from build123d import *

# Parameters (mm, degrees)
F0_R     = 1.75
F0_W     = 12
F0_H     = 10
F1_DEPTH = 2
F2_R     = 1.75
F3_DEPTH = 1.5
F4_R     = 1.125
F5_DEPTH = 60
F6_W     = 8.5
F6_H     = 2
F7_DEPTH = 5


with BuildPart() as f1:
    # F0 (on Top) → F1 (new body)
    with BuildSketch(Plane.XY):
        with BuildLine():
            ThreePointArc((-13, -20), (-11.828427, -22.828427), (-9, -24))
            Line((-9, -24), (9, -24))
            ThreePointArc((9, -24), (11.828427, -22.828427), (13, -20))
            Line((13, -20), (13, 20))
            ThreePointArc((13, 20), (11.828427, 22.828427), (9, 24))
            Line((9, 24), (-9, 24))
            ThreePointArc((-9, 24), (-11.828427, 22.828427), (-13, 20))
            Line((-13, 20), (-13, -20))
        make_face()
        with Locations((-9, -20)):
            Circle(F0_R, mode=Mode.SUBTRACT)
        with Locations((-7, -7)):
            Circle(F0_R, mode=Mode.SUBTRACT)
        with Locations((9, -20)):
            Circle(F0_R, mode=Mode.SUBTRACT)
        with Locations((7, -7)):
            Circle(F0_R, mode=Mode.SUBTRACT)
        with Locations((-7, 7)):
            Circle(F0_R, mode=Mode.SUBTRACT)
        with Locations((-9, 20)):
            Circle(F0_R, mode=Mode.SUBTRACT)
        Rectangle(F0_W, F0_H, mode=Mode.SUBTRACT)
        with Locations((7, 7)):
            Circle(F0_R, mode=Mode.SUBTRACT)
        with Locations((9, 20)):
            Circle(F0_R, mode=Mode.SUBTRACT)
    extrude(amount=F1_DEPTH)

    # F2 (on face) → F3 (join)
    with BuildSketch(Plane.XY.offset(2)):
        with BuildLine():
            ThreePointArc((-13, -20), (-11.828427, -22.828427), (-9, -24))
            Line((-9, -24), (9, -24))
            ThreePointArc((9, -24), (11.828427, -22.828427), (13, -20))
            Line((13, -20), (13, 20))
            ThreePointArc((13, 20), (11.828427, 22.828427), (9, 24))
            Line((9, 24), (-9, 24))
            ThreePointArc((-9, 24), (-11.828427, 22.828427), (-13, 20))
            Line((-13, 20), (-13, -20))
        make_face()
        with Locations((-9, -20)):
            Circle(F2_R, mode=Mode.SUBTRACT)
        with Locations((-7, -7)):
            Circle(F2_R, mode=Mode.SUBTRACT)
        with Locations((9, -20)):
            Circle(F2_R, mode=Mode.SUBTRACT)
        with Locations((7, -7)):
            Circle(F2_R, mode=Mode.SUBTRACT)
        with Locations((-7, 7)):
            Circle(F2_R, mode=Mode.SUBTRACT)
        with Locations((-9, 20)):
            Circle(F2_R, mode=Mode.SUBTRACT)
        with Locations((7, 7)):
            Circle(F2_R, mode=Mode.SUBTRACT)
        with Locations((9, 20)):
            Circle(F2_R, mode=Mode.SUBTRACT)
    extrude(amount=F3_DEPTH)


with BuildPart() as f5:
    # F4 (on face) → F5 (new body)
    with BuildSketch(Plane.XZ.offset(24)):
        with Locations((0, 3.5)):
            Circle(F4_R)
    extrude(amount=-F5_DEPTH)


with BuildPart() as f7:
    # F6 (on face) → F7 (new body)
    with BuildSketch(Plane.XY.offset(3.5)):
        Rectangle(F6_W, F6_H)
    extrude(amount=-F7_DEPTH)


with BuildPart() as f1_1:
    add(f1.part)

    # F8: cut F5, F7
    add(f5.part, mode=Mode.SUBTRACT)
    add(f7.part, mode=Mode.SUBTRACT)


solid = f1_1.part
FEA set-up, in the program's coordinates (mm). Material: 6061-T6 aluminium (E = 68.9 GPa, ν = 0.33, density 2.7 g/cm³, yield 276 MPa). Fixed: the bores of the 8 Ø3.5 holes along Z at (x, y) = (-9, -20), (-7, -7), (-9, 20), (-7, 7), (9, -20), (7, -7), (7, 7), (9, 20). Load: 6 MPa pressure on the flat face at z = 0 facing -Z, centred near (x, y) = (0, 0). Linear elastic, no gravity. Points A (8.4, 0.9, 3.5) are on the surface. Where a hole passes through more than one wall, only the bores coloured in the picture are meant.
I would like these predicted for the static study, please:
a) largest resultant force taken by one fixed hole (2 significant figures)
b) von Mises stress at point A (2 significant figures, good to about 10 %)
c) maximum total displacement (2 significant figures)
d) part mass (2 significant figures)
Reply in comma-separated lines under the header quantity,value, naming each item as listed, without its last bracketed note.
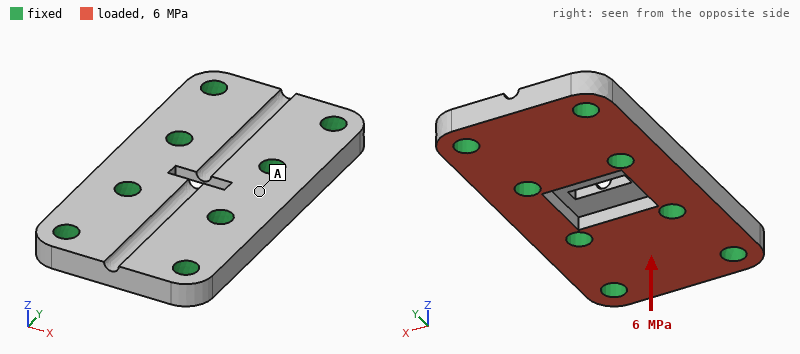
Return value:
quantity,value
largest resultant force taken by one fixed hole,840 N
von Mises stress at point A,15 MPa
maximum total displacement,9.0 µm
part mass,10.0 g
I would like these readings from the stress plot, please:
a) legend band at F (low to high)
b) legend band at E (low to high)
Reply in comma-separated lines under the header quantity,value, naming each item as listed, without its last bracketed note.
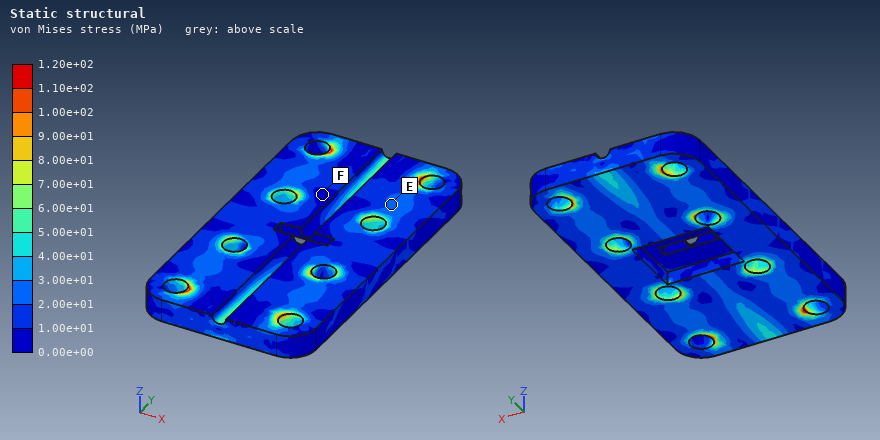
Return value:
quantity,value
legend band at F,0.00e+00 to 1.00e+01 MPa
legend band at E,2.00e+01 to 3.00e+01 MPa
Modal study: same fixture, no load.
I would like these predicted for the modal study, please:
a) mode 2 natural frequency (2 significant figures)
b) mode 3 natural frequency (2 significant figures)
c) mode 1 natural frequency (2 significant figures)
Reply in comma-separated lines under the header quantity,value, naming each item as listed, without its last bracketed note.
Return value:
quantity,value
mode 2 natural frequency,53 kHz
mode 3 natural frequency,64 kHz
mode 1 natural frequency,53 kHz
